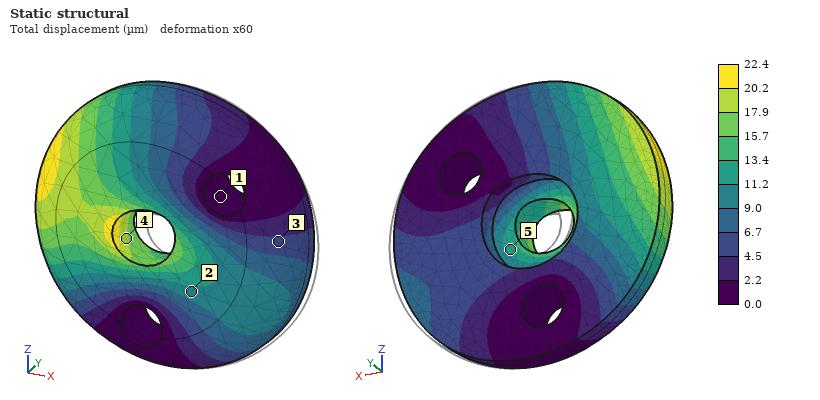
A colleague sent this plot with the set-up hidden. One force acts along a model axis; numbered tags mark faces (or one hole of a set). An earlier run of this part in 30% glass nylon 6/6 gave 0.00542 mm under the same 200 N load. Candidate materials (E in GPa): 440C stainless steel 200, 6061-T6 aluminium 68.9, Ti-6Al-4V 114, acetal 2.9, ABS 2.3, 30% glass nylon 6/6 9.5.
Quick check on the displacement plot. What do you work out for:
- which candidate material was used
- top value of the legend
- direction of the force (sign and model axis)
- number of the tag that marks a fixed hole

ABS
22.4 µm
-X
1
